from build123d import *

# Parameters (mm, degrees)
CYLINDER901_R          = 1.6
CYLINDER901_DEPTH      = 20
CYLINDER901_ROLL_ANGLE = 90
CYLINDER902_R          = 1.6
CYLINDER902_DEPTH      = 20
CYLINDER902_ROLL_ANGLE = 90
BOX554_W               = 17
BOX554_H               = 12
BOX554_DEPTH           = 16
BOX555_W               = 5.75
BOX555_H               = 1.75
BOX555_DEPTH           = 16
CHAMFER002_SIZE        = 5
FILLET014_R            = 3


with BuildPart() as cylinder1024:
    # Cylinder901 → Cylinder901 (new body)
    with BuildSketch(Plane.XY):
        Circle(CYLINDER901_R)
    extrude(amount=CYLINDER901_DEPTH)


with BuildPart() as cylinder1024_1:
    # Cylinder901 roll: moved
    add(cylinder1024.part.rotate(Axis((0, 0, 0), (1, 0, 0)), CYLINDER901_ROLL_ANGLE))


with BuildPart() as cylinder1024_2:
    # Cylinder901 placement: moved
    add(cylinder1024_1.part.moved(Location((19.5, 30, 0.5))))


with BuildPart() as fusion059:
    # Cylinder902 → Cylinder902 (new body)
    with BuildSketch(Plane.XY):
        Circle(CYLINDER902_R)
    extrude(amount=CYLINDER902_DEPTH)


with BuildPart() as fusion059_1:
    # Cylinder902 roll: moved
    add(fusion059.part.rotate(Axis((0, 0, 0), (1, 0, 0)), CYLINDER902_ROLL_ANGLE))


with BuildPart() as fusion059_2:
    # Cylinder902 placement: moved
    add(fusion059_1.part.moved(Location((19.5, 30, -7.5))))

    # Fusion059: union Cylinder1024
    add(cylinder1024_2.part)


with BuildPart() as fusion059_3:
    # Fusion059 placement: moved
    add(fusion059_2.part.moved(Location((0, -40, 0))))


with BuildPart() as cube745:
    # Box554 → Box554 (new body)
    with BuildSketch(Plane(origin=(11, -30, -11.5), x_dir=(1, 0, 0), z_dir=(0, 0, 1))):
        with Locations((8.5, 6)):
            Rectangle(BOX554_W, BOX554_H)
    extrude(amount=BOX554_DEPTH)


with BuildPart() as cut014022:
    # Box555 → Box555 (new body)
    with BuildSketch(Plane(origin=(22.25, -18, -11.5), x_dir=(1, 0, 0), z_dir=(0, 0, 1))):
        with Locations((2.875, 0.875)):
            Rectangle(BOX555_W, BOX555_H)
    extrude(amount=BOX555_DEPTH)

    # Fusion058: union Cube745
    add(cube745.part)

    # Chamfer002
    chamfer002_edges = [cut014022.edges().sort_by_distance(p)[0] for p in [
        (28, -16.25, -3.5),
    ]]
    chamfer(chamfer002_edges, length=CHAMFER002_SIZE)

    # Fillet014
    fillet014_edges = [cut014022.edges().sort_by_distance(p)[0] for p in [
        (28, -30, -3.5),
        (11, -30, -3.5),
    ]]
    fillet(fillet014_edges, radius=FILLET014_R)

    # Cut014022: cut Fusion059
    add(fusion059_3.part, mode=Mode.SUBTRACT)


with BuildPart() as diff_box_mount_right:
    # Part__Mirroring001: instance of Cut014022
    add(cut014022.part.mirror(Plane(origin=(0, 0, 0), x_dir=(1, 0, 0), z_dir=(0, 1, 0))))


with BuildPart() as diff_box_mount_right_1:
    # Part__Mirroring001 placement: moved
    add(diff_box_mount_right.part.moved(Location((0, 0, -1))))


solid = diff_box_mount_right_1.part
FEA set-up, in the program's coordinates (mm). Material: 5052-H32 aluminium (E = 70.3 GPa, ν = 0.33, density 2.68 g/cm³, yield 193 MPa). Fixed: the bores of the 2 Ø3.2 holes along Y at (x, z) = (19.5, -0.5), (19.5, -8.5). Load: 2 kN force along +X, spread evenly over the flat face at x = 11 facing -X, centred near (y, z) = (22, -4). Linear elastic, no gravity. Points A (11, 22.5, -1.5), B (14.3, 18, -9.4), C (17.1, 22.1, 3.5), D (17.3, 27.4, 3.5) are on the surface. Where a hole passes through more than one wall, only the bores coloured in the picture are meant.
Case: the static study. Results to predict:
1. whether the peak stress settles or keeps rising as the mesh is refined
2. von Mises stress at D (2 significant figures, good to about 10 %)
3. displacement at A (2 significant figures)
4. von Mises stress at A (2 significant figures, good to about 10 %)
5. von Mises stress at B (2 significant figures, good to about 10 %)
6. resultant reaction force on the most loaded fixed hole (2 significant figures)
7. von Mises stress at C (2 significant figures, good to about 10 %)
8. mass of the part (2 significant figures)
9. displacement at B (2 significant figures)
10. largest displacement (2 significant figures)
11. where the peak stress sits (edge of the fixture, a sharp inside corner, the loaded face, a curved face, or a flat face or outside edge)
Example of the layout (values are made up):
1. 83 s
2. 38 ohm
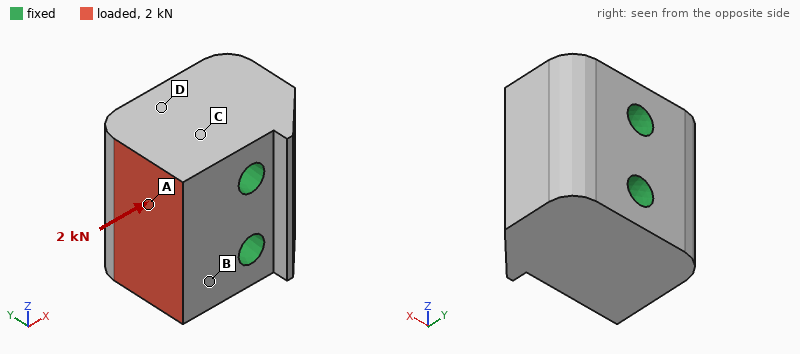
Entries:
1. keeps rising
2. 5.5 MPa
3. 1.6 µm
4. 14 MPa
5. 16 MPa
6. 1.0 kN
7. 8.6 MPa
8. 8.0 g
9. 1.3 µm
10. 2.2 µm
11. edge of the fixture
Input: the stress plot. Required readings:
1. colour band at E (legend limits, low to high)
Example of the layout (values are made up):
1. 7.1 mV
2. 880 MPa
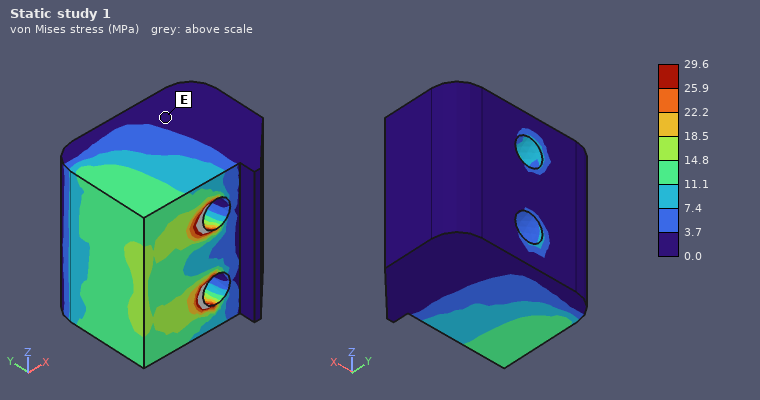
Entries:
1. 0.0 to 3.7 MPa
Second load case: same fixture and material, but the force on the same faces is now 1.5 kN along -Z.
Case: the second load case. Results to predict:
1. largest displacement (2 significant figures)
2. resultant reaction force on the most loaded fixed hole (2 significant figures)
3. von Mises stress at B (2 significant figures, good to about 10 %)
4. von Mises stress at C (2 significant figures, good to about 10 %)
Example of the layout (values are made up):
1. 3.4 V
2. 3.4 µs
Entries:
1. 6.3 µm
2. 1.4 kN
3. 16 MPa
4. 19 MPa
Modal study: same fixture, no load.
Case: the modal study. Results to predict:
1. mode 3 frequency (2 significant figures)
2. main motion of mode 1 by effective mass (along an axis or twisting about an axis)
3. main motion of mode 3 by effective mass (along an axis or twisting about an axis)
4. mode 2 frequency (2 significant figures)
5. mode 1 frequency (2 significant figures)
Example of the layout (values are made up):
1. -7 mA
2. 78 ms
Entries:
1. 86 kHz
2. twisting about Y
3. along Y
4. 80 kHz
5. 76 kHz
